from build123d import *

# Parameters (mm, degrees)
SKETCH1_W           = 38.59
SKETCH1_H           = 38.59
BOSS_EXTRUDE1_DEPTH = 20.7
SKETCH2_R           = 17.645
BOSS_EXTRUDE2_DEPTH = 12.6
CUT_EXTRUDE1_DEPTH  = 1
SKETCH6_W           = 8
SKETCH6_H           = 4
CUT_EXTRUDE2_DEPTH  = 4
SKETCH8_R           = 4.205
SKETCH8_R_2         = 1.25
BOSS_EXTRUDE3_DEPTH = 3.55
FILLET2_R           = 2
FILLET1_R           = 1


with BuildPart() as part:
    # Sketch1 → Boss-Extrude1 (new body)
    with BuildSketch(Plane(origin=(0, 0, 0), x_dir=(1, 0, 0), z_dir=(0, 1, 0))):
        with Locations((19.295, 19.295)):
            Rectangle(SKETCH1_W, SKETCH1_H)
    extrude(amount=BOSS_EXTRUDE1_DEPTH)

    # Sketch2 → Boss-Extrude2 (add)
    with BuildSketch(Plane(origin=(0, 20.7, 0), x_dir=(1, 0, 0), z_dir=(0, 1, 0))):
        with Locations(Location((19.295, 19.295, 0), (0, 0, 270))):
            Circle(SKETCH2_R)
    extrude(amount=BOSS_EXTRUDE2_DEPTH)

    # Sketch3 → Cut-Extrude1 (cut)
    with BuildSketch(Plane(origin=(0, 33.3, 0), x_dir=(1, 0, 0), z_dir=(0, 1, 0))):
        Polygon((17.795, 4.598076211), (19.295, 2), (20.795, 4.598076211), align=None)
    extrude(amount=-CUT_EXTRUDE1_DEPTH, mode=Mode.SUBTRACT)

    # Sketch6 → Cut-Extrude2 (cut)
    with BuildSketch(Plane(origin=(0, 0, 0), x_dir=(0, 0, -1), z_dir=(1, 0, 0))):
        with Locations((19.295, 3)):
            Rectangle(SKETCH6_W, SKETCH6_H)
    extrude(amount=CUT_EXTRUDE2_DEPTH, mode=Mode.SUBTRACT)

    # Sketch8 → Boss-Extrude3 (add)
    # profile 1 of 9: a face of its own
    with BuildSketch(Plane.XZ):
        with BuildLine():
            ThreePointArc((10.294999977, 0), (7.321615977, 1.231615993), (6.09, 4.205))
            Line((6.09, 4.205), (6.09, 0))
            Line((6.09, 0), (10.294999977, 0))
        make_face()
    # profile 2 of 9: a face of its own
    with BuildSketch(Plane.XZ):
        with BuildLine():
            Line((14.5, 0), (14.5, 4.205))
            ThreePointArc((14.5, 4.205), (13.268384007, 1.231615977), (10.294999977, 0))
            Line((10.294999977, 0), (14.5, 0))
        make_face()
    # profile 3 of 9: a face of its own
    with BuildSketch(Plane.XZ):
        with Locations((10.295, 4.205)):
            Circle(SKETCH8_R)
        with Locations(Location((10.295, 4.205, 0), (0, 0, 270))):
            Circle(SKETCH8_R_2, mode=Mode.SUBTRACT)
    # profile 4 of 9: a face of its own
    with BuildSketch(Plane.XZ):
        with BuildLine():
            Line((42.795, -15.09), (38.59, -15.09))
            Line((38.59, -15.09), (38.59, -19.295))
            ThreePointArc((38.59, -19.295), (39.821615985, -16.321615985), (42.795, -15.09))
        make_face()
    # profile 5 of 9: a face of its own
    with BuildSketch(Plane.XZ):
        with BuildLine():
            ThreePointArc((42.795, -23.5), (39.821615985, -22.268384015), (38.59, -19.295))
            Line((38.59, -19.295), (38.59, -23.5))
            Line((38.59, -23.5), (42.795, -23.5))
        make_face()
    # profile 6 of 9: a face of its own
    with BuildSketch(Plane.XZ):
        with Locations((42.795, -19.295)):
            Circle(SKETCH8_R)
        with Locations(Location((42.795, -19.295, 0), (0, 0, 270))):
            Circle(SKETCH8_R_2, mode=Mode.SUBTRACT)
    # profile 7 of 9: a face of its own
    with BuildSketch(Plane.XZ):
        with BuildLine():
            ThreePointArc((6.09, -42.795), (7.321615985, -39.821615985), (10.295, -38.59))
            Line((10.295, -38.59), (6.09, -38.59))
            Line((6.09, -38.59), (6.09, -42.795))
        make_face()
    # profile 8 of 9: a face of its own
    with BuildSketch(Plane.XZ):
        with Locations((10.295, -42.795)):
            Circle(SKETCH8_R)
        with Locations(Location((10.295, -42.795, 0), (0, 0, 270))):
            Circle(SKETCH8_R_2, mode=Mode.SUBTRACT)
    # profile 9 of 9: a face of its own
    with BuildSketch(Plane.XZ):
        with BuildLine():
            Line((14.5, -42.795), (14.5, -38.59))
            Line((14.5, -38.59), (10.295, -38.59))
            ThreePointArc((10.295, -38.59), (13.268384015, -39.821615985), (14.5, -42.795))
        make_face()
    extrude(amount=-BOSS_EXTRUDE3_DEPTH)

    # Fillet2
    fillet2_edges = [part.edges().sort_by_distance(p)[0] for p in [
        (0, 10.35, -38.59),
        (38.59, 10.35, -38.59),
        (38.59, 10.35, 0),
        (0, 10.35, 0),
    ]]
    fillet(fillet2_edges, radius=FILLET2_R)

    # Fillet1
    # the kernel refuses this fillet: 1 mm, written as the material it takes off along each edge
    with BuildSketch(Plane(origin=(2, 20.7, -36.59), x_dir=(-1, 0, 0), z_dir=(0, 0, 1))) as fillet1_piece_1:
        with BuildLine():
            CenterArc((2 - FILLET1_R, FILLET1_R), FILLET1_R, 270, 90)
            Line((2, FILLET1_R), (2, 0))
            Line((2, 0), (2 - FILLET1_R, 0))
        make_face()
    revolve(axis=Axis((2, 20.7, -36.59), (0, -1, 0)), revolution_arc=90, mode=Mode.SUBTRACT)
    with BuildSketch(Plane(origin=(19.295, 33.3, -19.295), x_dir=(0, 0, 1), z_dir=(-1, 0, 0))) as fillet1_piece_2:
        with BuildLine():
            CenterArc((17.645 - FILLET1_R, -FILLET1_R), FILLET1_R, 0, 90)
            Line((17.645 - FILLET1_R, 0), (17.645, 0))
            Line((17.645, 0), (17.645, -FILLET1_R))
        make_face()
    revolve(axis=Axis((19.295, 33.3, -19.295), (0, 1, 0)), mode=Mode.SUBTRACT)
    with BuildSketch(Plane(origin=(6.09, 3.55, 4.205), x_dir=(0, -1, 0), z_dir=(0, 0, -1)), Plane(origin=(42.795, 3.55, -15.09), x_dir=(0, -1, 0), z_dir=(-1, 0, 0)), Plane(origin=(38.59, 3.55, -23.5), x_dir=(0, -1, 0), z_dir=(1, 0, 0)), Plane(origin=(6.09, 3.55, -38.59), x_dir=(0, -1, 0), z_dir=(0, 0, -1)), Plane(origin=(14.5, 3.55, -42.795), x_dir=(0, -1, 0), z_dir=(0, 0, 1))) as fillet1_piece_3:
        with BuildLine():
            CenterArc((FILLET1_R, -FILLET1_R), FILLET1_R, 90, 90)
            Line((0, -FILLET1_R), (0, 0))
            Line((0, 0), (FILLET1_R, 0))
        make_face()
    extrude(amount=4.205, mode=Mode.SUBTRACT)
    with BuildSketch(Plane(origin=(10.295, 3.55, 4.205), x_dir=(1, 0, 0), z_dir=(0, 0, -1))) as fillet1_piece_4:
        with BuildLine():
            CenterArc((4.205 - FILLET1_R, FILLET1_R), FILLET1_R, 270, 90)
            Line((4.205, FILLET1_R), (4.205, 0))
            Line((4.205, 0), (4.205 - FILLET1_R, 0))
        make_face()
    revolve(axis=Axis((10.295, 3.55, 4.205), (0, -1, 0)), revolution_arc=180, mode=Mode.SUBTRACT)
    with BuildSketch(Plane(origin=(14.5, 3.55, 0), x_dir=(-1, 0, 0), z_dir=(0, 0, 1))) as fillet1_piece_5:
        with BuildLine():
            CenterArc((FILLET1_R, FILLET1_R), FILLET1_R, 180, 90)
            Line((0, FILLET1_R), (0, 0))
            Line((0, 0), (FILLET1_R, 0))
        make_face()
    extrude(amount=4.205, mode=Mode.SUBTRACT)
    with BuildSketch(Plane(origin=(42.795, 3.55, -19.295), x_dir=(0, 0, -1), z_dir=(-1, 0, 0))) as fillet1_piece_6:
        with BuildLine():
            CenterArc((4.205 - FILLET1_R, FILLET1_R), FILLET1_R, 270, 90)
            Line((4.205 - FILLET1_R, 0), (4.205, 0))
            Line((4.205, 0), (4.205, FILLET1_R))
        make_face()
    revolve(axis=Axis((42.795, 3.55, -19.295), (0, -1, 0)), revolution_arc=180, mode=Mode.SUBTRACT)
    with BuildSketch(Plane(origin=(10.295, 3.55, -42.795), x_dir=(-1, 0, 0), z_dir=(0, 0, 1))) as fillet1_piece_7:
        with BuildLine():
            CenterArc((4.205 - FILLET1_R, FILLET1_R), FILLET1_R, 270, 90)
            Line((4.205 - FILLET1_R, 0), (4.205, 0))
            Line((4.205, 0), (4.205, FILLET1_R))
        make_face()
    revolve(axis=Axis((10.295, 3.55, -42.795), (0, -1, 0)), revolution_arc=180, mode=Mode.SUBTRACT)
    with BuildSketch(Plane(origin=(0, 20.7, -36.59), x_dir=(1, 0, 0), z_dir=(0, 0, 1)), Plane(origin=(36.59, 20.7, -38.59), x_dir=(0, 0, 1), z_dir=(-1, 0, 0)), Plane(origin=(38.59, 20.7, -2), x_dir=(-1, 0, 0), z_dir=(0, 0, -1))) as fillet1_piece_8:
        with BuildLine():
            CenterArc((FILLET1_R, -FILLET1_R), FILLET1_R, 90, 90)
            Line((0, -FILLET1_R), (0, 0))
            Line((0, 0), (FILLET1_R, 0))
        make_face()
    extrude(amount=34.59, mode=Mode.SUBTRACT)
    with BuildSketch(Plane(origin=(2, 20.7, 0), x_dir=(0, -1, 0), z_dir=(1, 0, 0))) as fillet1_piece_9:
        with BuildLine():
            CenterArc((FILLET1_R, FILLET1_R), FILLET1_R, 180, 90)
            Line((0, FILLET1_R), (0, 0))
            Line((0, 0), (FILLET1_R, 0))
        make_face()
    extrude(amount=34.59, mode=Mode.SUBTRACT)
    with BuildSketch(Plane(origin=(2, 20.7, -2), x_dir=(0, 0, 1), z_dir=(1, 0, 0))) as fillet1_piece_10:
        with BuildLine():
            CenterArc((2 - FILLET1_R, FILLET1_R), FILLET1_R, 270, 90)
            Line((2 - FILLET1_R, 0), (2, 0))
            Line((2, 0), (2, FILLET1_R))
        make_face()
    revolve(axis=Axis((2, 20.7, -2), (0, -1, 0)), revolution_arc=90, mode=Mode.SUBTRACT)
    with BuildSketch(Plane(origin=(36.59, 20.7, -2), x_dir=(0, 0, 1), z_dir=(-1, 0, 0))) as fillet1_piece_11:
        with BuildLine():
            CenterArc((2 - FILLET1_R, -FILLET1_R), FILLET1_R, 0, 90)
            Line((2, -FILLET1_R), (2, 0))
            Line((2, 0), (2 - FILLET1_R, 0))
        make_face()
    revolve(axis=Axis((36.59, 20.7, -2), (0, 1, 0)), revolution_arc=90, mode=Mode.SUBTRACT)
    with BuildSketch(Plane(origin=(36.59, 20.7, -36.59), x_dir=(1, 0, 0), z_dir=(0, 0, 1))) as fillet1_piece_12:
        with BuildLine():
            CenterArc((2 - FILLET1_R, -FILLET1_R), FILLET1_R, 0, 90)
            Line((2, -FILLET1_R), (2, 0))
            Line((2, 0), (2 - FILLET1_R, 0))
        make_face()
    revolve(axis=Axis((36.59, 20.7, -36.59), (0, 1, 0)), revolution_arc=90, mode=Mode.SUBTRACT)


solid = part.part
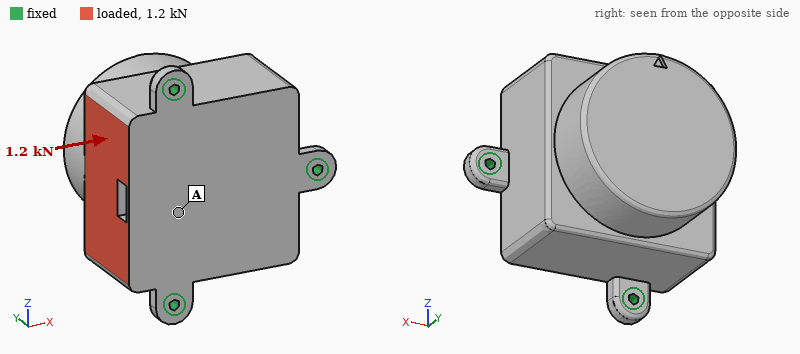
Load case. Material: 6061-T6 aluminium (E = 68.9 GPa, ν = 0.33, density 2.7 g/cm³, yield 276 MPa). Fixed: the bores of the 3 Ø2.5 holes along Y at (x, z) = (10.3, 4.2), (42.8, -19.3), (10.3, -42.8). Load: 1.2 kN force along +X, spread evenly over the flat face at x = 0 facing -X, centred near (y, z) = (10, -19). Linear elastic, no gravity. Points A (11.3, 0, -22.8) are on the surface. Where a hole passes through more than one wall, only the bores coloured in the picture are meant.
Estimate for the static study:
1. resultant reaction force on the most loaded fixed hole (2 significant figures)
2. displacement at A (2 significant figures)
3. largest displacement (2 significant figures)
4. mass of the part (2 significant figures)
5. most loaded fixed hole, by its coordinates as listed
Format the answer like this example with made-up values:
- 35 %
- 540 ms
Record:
- 760 N
- 3.6 µm
- 11 µm
- 120 g
- (42.8, -19.3)
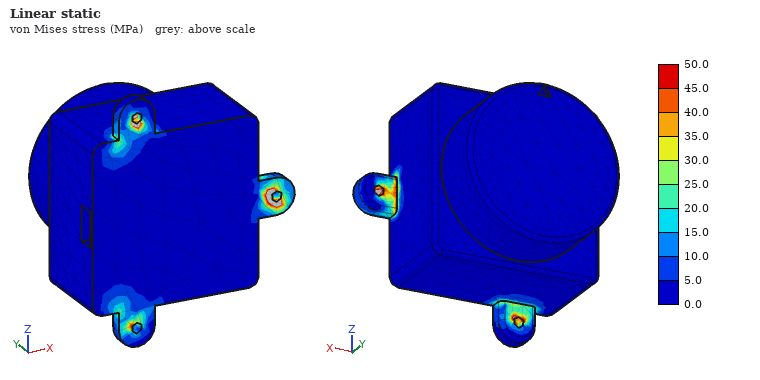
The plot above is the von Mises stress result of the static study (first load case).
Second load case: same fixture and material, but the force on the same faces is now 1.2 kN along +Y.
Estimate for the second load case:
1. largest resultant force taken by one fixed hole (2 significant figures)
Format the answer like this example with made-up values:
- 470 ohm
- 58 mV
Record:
- 880 N
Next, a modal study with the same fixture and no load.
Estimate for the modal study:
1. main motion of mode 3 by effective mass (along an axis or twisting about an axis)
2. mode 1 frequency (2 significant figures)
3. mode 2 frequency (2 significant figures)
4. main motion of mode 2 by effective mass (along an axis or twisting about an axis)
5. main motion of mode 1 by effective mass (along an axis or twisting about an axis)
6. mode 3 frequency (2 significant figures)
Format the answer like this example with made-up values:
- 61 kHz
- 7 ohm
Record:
- along Y
- 4500 Hz
- 5400 Hz
- along Z
- along X
- 6400 Hz
